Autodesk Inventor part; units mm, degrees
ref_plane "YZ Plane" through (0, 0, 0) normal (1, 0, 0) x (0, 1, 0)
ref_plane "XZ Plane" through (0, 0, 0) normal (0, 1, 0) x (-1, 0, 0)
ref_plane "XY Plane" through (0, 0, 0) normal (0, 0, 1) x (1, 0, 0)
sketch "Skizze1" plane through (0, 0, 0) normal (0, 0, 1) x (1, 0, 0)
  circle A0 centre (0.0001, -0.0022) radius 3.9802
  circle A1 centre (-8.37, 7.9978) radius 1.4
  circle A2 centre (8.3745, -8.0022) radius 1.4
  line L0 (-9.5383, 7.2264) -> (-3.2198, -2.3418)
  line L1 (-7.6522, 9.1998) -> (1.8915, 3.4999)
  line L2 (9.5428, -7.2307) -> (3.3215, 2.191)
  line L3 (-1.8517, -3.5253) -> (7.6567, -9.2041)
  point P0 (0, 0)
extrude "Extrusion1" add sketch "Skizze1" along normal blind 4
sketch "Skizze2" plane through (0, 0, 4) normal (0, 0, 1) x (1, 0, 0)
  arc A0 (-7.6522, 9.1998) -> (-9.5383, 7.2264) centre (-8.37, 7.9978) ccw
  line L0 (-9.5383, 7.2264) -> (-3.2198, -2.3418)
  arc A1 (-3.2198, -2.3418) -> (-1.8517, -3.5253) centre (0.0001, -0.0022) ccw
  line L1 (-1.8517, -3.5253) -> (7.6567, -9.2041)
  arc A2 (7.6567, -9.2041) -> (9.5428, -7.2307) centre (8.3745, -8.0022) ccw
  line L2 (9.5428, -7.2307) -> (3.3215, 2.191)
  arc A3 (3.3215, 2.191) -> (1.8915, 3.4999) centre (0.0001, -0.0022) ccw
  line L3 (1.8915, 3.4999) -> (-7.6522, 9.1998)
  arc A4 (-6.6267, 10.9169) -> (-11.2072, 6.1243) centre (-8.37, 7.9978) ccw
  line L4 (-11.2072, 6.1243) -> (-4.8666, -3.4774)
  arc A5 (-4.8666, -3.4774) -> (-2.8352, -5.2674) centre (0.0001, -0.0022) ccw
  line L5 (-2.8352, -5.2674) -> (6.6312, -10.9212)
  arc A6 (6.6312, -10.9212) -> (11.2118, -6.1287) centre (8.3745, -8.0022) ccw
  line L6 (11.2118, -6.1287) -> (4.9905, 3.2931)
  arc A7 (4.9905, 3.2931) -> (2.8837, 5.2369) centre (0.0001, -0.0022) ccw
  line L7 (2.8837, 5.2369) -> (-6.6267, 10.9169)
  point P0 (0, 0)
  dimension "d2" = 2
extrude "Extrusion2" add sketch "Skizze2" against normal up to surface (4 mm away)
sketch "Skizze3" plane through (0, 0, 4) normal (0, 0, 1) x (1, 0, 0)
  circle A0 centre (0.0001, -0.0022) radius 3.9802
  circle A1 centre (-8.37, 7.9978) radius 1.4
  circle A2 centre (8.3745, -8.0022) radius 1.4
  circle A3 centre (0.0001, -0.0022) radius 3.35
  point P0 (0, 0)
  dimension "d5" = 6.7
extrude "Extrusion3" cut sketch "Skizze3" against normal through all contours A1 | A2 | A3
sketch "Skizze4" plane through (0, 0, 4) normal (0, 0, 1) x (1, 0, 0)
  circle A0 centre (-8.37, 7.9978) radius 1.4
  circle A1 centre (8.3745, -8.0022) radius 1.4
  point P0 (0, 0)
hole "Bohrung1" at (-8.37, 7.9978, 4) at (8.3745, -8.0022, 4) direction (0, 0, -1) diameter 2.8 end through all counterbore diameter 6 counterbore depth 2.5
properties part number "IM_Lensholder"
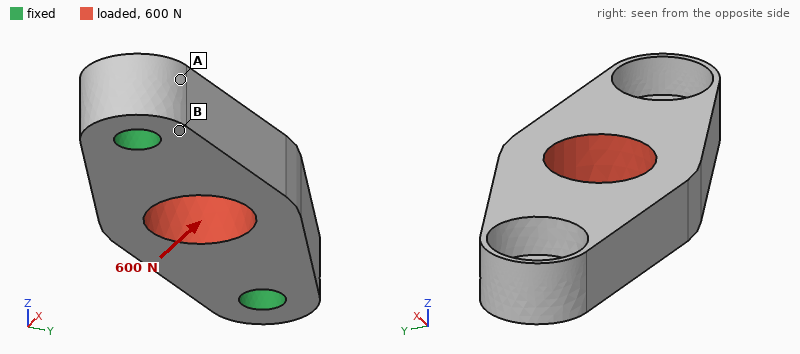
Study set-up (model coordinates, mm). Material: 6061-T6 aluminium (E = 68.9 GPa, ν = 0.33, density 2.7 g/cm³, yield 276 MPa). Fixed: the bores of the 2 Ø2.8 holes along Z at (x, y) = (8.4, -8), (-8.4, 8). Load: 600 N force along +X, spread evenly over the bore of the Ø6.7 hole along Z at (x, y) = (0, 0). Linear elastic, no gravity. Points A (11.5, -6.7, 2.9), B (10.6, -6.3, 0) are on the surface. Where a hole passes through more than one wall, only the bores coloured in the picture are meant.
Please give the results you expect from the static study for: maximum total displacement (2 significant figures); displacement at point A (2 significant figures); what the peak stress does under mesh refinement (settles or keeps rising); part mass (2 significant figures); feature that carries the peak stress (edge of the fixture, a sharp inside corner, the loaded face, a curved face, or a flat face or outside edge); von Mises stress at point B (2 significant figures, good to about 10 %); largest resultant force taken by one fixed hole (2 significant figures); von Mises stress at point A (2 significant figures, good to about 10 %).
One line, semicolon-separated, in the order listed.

13 µm; 2.4 µm; keeps rising; 2.0 g; edge of the fixture; 34 MPa; 300 N; 16 MPa
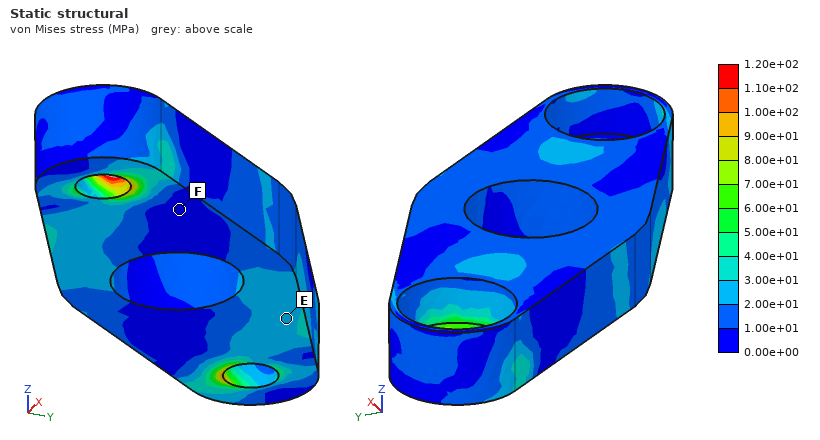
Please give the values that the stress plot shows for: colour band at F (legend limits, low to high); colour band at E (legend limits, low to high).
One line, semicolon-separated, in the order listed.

0.00e+00 to 1.00e+01 MPa; 2.00e+01 to 3.00e+01 MPa
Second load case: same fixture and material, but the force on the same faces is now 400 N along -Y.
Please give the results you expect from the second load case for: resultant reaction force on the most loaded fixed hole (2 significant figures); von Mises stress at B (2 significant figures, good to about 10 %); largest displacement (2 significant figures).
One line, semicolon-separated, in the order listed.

200 N; 16 MPa; 8.7 µm
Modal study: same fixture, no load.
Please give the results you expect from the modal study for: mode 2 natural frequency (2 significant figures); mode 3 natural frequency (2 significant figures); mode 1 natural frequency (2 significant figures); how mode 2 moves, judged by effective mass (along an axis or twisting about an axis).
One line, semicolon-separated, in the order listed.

22 kHz; 43 kHz; 20 kHz; along Z
